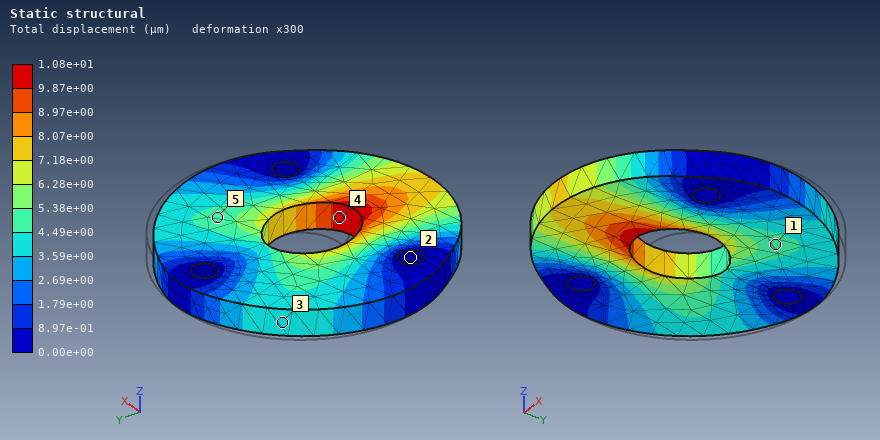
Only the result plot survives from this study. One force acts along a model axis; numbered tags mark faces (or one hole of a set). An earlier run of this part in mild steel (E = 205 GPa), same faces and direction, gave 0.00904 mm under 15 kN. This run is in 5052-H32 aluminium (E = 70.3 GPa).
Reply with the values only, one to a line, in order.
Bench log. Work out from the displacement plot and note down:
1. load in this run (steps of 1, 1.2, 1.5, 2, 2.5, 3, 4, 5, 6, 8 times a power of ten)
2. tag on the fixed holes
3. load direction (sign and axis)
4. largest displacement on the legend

6 kN
2
-Y
1.08e+01 µm
